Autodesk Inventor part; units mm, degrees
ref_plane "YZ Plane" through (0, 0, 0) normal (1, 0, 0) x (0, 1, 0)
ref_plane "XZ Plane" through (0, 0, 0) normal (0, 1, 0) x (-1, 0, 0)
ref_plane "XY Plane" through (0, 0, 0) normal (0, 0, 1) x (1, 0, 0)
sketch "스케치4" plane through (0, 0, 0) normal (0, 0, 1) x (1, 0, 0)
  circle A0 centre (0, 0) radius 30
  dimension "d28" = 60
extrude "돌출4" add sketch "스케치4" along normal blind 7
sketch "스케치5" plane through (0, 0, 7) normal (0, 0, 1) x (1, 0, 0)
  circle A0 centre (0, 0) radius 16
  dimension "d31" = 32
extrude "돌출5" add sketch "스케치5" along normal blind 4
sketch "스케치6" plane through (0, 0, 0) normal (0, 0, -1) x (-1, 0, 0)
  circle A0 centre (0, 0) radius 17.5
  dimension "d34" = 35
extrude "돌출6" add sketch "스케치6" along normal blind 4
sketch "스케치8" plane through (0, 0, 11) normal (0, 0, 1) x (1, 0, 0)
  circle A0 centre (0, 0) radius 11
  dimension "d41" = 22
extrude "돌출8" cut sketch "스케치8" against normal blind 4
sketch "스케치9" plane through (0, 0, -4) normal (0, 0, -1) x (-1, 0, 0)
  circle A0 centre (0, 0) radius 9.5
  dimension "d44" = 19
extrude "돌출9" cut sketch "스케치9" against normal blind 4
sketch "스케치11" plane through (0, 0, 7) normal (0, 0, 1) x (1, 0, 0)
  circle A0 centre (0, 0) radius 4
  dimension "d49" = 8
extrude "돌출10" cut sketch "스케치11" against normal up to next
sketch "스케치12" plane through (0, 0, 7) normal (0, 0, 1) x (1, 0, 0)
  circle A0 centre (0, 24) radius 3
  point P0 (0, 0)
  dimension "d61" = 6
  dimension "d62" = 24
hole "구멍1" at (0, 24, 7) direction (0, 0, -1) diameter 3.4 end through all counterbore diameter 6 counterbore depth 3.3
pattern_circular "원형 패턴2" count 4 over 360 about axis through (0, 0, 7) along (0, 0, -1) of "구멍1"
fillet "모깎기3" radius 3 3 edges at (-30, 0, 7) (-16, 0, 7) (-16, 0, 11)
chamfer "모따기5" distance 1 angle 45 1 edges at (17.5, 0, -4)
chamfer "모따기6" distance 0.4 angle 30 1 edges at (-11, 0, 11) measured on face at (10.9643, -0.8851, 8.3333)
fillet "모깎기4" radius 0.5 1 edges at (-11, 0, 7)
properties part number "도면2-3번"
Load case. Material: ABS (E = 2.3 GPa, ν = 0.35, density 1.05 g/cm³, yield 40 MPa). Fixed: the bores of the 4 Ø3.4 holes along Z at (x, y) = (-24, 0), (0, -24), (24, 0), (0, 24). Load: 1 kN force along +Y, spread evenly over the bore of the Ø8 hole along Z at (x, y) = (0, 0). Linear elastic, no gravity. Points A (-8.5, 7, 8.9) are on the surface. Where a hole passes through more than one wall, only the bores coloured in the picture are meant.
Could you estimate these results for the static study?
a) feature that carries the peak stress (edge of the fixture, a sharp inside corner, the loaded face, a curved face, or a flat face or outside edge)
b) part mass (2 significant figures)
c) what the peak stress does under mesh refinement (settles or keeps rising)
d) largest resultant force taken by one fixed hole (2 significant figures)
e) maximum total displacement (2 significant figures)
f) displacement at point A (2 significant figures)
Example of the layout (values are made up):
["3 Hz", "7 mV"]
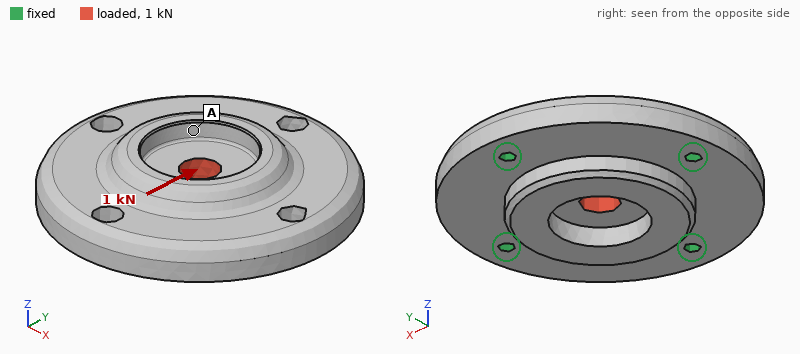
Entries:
["edge of the fixture", "24 g", "keeps rising", "310 N", "44 µm", "24 µm"]
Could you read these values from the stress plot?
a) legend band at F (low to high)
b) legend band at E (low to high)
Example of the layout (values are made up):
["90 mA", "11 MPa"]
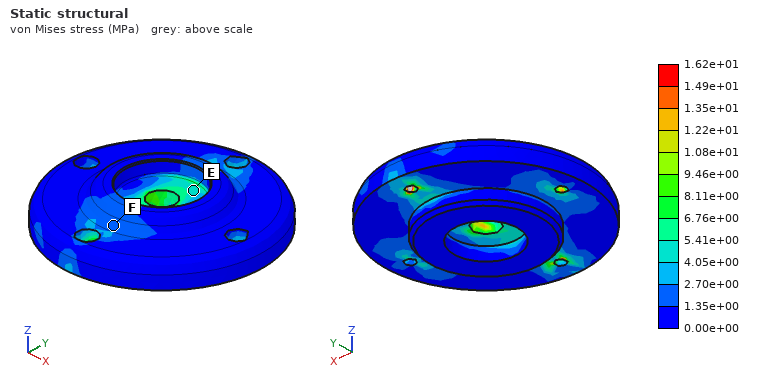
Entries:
["1.35e+00 to 2.70e+00 MPa", "4.05e+00 to 5.41e+00 MPa"]
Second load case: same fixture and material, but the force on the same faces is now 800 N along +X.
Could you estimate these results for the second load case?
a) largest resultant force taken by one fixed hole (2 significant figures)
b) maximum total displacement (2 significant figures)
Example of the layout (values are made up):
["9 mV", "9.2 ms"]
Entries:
["250 N", "35 µm"]
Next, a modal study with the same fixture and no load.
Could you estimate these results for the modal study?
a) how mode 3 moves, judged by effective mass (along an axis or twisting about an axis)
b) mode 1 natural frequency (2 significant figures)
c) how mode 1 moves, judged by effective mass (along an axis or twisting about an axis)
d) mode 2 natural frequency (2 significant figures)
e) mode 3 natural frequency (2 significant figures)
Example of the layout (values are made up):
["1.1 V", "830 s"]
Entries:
["twisting about Y", "4700 Hz", "along Z", "4900 Hz", "5200 Hz"]
